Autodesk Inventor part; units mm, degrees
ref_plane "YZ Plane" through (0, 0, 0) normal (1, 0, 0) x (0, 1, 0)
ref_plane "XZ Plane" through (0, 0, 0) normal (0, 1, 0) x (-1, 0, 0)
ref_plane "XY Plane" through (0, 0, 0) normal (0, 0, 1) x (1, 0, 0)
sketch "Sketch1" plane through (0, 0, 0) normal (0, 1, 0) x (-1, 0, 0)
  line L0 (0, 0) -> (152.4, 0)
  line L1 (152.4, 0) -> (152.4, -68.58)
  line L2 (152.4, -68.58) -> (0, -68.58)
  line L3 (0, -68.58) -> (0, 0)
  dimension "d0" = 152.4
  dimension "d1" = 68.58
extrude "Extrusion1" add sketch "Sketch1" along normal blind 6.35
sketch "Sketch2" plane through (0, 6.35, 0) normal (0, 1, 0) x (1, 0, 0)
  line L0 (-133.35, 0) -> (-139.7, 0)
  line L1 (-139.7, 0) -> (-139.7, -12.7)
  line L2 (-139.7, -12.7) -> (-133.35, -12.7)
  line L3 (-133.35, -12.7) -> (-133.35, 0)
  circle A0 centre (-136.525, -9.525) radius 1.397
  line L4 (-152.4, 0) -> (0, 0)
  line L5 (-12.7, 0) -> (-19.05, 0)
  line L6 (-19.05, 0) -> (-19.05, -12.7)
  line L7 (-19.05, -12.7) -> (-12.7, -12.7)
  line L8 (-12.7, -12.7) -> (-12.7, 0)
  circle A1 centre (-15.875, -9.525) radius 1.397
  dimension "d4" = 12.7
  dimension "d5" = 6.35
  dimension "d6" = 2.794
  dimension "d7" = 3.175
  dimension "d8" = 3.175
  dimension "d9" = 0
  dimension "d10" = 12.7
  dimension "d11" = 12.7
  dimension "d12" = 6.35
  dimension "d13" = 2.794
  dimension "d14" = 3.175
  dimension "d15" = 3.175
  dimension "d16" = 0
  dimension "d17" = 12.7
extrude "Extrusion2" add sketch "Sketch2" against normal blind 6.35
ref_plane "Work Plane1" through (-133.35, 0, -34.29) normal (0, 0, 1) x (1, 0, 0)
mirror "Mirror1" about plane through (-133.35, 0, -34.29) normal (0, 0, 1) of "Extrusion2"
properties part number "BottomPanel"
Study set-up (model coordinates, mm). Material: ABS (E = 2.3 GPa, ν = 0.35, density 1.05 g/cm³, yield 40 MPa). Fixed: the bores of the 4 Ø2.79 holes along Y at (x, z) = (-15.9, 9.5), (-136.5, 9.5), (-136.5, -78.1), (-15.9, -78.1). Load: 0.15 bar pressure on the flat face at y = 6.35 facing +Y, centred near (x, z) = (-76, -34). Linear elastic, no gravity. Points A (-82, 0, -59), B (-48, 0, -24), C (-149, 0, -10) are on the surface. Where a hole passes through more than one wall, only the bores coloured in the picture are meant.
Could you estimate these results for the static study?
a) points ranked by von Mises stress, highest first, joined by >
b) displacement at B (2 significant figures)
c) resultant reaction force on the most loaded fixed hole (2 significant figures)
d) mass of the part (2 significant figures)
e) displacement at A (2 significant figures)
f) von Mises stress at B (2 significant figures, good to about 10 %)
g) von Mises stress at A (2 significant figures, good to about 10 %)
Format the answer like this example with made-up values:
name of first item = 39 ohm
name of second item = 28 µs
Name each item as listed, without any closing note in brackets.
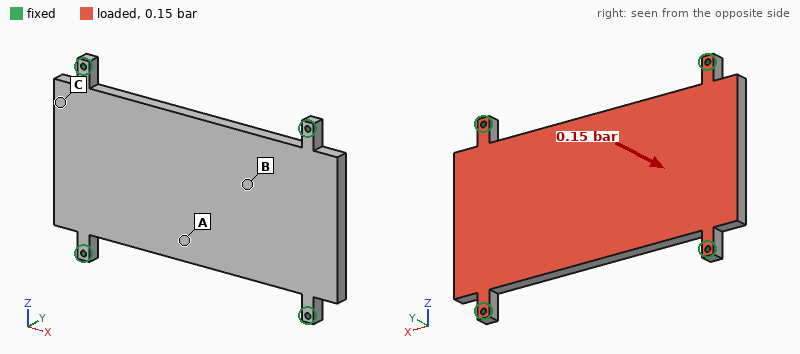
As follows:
points ranked by von Mises stress, highest first, joined by > = A > B > C
displacement at B = 0.49 mm
resultant reaction force on the most loaded fixed hole = 40 N
mass of the part = 72 g
displacement at A = 0.61 mm
von Mises stress at B = 1.7 MPa
von Mises stress at A = 2.8 MPa
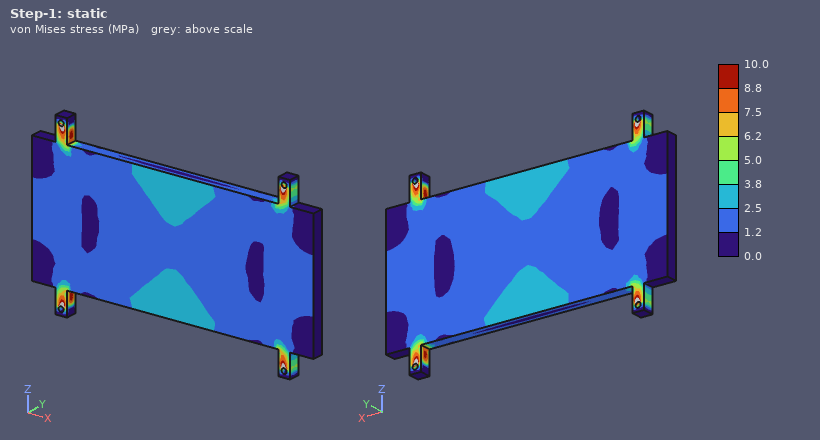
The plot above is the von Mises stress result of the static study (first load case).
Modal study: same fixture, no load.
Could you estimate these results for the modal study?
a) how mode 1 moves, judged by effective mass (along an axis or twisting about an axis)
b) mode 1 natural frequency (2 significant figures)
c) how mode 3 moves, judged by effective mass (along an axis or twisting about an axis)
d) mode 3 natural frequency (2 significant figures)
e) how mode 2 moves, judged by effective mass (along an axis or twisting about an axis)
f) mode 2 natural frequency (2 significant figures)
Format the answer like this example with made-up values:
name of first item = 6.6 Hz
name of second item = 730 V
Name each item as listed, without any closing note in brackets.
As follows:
how mode 1 moves, judged by effective mass = along Y
mode 1 natural frequency = 340 Hz
how mode 3 moves, judged by effective mass = twisting about Z
mode 3 natural frequency = 830 Hz
how mode 2 moves, judged by effective mass = twisting about X
mode 2 natural frequency = 790 Hz
